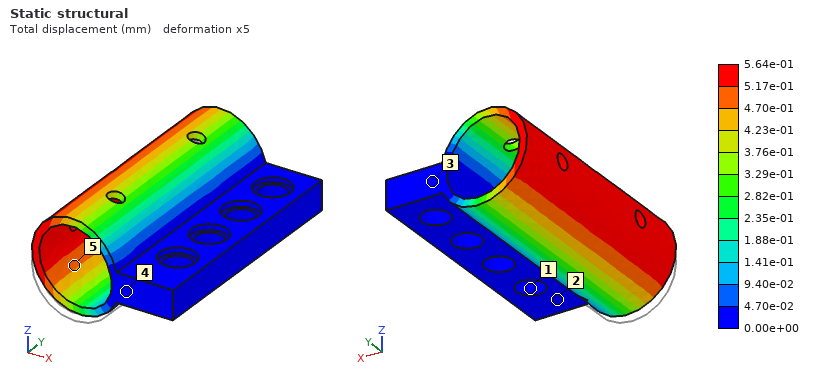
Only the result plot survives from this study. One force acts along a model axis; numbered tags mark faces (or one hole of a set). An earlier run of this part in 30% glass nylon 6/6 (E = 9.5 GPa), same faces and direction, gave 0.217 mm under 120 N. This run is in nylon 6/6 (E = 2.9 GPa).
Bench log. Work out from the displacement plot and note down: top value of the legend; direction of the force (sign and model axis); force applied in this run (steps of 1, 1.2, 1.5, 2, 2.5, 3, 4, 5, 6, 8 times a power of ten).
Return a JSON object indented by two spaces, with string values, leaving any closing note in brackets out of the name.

{
  "top value of the legend": "5.64e-01 mm",
  "direction of the force": "+Z",
  "force applied in this run": "100 N"
}
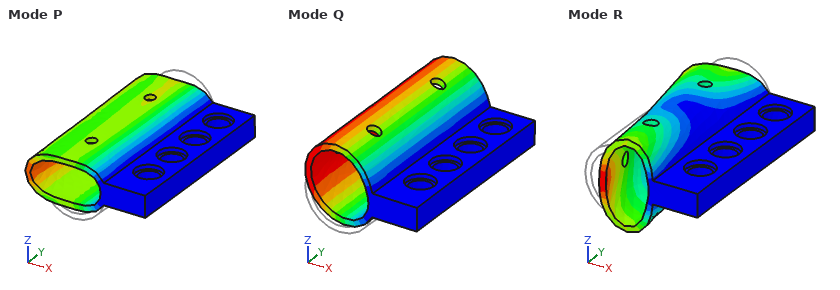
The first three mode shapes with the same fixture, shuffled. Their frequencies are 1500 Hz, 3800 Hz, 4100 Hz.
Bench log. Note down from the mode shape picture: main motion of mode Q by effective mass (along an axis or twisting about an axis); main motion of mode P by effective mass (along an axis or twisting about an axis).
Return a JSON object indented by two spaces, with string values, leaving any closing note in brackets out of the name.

{
  "main motion of mode Q by effective mass": "along Z",
  "main motion of mode P by effective mass": "along X"
}
